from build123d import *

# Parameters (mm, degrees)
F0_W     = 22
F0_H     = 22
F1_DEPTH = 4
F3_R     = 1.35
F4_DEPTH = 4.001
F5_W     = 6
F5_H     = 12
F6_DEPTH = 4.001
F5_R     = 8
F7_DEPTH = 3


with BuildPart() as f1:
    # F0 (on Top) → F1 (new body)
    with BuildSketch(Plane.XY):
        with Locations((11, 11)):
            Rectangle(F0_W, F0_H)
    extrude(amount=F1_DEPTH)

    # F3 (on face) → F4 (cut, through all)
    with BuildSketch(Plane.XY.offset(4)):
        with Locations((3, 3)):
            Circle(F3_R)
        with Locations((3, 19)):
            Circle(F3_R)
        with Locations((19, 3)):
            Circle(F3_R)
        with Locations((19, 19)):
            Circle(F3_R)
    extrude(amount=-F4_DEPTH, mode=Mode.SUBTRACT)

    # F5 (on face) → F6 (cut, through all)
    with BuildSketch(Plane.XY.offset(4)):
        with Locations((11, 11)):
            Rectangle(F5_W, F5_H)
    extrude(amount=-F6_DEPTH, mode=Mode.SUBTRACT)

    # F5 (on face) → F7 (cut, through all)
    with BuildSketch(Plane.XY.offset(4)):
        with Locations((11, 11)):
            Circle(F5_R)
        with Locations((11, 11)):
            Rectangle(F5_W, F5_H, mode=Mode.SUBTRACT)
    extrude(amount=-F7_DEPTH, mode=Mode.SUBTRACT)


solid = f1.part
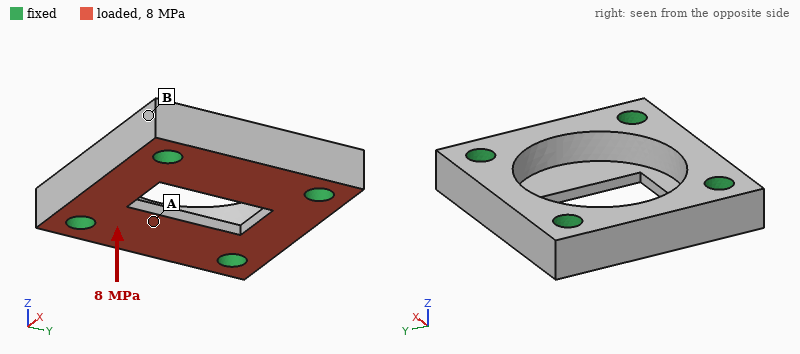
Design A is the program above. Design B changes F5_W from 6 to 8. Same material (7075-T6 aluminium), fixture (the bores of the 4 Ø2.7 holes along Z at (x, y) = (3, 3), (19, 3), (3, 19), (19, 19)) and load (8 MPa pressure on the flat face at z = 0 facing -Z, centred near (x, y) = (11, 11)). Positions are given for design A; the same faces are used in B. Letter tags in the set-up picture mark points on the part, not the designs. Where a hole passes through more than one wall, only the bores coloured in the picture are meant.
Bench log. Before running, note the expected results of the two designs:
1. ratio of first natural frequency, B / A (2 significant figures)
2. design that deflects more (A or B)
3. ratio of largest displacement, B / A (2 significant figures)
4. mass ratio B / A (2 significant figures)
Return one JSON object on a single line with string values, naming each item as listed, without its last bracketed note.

{"ratio of first natural frequency, B / A": "1.3", "design that deflects more": "A", "ratio of largest displacement, B / A": "0.60", "mass ratio B / A": "0.98"}
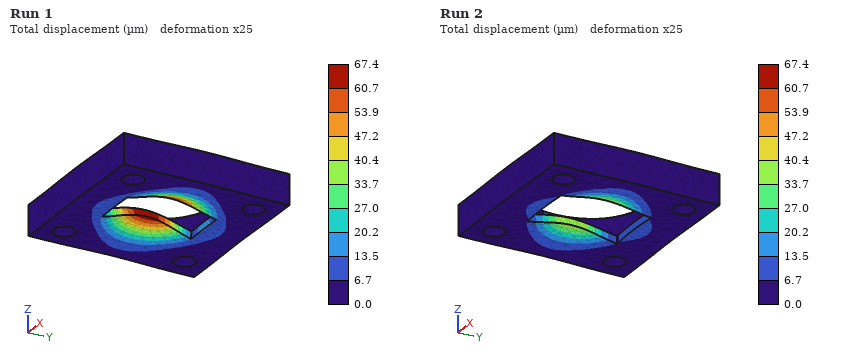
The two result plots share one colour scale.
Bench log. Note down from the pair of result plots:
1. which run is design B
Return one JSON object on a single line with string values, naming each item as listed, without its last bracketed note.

{"which run is design B": "Run 2"}
